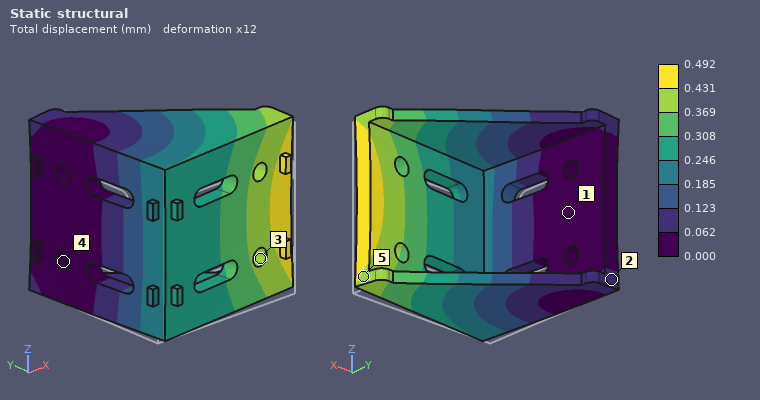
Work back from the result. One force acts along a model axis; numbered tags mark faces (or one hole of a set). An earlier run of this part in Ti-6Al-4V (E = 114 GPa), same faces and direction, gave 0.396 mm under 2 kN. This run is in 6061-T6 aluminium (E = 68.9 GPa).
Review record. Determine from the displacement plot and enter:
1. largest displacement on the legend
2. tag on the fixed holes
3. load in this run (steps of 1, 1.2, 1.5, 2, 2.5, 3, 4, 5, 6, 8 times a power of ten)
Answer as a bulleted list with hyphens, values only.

- 0.492 mm
- 4
- 1.5 kN
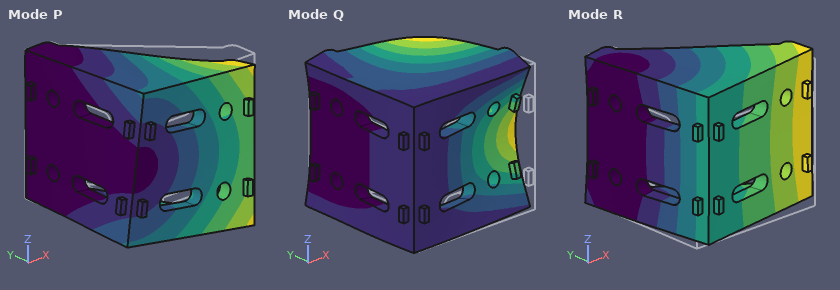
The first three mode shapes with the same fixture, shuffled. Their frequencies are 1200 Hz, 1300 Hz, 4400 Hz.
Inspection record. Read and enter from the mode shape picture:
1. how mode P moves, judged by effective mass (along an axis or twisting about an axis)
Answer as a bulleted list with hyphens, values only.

- along Z
